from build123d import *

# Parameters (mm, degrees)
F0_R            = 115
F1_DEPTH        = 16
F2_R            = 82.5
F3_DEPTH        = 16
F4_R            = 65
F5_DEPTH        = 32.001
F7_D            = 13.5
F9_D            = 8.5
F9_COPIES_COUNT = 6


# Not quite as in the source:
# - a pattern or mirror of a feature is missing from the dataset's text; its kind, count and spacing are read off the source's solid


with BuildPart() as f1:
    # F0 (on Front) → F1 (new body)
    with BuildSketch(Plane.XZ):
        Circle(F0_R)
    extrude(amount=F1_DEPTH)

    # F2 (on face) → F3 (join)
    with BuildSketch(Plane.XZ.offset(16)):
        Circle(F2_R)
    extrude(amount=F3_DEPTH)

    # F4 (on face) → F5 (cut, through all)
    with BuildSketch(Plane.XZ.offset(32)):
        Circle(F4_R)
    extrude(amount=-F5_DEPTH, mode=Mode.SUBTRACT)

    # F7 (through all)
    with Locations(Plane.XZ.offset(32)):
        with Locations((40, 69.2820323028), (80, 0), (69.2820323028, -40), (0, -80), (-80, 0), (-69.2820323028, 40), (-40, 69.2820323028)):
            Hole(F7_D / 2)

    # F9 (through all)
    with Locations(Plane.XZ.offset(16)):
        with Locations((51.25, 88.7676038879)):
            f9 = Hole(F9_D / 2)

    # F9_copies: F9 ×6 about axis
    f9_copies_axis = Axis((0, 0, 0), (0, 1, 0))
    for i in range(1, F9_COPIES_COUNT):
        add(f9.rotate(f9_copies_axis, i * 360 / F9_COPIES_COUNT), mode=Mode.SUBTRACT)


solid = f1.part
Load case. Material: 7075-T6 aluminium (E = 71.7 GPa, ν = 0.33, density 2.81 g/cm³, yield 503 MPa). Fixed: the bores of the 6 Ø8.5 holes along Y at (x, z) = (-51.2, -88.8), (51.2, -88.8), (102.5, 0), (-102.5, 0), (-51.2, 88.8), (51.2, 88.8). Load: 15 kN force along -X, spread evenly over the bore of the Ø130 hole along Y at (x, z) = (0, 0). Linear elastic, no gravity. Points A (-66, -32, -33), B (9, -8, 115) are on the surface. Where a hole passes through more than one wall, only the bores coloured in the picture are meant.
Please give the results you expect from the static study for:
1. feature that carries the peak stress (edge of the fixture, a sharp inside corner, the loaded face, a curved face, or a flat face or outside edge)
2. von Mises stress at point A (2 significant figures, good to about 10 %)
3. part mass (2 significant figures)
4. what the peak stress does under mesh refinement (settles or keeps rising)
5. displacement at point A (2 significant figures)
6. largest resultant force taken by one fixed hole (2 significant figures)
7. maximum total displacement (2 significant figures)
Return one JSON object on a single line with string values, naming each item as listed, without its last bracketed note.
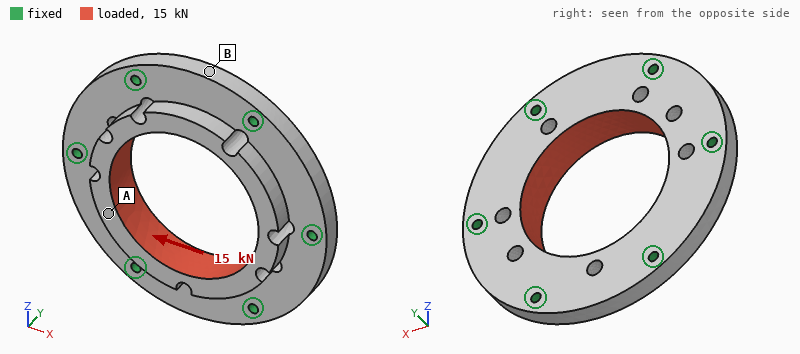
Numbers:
{"feature that carries the peak stress": "a sharp inside corner", "von Mises stress at point A": "2.5 MPa", "part mass": "1.5 kg", "what the peak stress does under mesh refinement": "keeps rising", "displacement at point A": "6.2 µm", "largest resultant force taken by one fixed hole": "2.9 kN", "maximum total displacement": "7.8 µm"}
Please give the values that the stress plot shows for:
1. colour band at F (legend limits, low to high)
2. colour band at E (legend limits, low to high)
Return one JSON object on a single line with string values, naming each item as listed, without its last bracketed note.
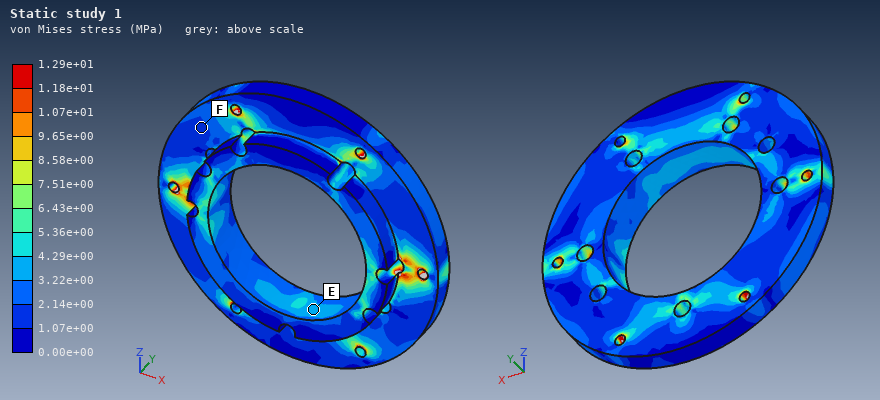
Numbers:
{"colour band at F": "1.07e+00 to 2.14e+00 MPa", "colour band at E": "3.22e+00 to 4.29e+00 MPa"}
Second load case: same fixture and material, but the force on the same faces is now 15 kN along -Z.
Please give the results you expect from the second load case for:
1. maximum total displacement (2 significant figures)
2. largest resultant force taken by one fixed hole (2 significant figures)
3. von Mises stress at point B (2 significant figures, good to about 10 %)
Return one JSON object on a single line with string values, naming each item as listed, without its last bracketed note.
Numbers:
{"maximum total displacement": "8.5 µm", "largest resultant force taken by one fixed hole": "2.9 kN", "von Mises stress at point B": "2.8 MPa"}
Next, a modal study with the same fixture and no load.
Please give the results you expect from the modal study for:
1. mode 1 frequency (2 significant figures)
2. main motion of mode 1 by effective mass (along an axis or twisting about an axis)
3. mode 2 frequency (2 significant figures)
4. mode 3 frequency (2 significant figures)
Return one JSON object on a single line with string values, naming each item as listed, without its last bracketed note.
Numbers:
{"mode 1 frequency": "5100 Hz", "main motion of mode 1 by effective mass": "along Y", "mode 2 frequency": "6000 Hz", "mode 3 frequency": "6000 Hz"}
